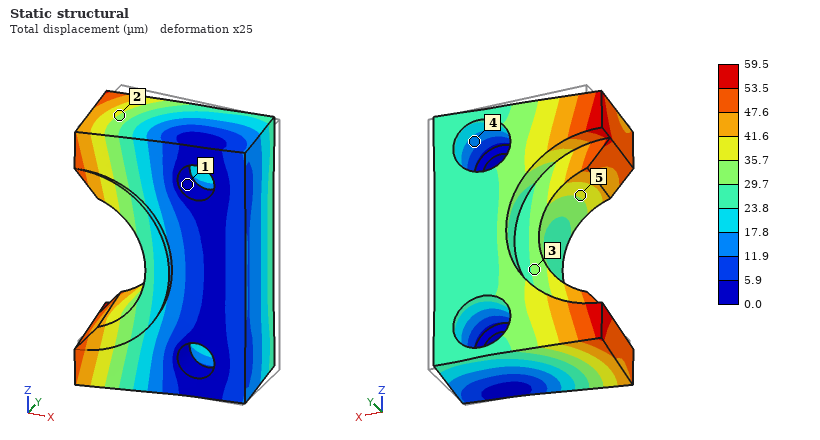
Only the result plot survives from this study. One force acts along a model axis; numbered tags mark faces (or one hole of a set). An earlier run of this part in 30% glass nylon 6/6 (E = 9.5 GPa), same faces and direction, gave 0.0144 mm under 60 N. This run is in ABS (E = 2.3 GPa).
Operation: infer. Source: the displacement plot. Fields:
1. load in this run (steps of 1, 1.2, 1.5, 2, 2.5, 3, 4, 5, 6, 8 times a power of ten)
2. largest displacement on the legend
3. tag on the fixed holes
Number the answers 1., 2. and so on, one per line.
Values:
1. 60 N
2. 59.5 µm
3. 1
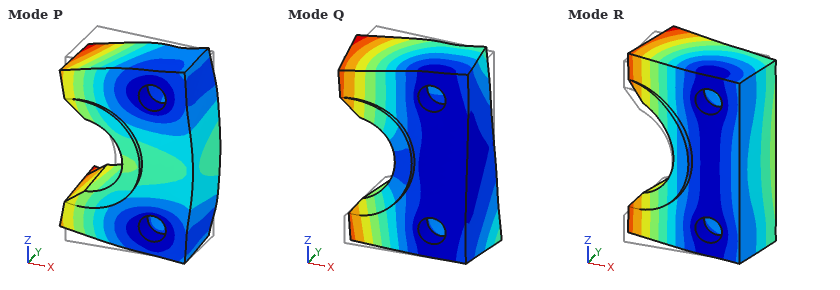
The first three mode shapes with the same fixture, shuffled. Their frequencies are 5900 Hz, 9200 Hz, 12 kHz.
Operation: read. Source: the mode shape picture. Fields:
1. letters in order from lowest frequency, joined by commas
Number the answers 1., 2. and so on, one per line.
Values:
1. R, Q, P
